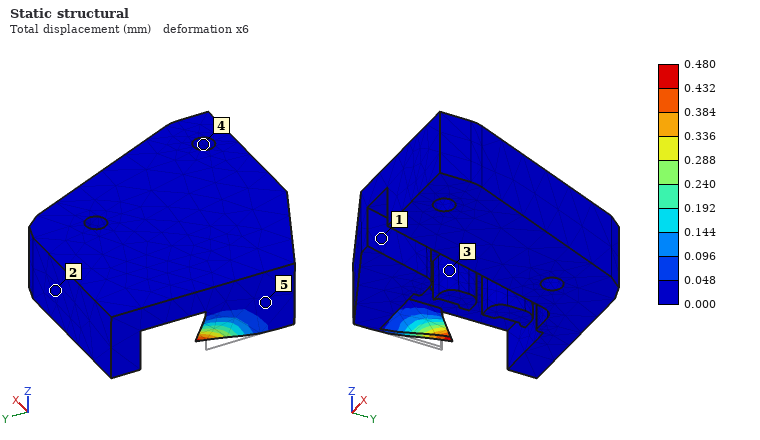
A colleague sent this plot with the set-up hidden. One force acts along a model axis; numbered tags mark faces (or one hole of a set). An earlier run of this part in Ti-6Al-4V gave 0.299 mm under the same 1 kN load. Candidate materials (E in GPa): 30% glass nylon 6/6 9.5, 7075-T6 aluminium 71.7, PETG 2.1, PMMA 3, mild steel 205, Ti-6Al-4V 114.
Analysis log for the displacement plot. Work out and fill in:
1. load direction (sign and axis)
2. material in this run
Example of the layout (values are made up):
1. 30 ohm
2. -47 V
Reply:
1. +X
2. 7075-T6 aluminium
